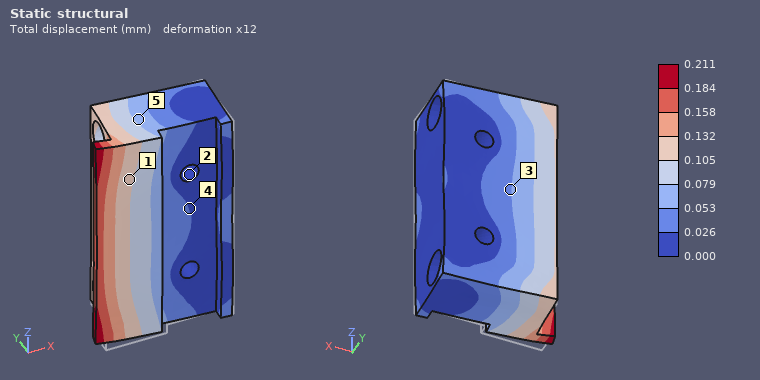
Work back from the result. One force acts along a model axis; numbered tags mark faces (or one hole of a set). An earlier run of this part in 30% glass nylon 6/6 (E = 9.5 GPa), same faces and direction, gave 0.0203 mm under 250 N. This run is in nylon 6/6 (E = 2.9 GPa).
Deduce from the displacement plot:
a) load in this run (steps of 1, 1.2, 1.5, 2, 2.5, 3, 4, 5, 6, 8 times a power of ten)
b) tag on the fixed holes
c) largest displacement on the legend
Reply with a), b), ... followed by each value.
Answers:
a) 800 N
b) 2
c) 0.211 mm
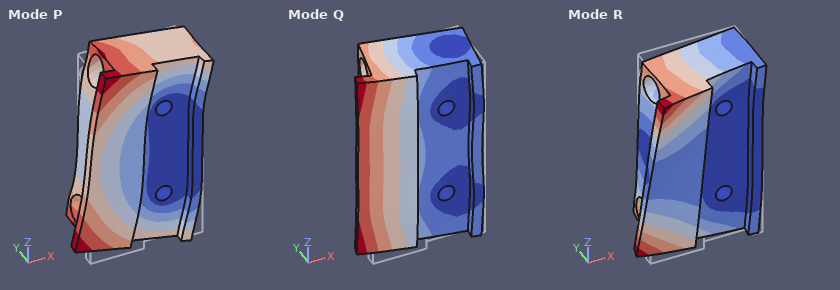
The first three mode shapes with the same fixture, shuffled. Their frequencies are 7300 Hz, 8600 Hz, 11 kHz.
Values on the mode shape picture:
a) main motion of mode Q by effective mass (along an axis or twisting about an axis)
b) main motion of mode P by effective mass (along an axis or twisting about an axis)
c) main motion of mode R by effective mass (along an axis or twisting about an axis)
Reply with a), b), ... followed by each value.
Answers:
a) along Y
b) along Z
c) twisting about X
